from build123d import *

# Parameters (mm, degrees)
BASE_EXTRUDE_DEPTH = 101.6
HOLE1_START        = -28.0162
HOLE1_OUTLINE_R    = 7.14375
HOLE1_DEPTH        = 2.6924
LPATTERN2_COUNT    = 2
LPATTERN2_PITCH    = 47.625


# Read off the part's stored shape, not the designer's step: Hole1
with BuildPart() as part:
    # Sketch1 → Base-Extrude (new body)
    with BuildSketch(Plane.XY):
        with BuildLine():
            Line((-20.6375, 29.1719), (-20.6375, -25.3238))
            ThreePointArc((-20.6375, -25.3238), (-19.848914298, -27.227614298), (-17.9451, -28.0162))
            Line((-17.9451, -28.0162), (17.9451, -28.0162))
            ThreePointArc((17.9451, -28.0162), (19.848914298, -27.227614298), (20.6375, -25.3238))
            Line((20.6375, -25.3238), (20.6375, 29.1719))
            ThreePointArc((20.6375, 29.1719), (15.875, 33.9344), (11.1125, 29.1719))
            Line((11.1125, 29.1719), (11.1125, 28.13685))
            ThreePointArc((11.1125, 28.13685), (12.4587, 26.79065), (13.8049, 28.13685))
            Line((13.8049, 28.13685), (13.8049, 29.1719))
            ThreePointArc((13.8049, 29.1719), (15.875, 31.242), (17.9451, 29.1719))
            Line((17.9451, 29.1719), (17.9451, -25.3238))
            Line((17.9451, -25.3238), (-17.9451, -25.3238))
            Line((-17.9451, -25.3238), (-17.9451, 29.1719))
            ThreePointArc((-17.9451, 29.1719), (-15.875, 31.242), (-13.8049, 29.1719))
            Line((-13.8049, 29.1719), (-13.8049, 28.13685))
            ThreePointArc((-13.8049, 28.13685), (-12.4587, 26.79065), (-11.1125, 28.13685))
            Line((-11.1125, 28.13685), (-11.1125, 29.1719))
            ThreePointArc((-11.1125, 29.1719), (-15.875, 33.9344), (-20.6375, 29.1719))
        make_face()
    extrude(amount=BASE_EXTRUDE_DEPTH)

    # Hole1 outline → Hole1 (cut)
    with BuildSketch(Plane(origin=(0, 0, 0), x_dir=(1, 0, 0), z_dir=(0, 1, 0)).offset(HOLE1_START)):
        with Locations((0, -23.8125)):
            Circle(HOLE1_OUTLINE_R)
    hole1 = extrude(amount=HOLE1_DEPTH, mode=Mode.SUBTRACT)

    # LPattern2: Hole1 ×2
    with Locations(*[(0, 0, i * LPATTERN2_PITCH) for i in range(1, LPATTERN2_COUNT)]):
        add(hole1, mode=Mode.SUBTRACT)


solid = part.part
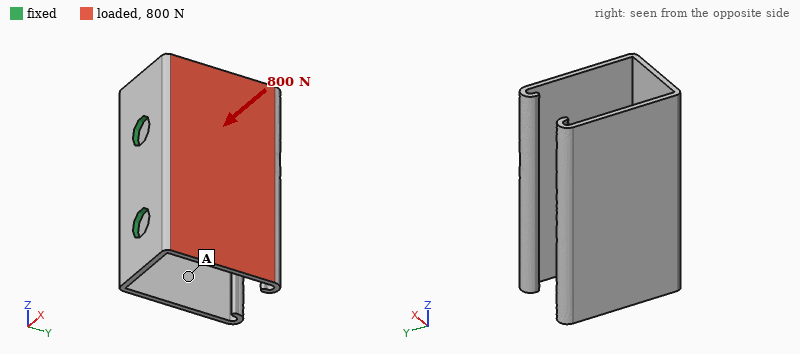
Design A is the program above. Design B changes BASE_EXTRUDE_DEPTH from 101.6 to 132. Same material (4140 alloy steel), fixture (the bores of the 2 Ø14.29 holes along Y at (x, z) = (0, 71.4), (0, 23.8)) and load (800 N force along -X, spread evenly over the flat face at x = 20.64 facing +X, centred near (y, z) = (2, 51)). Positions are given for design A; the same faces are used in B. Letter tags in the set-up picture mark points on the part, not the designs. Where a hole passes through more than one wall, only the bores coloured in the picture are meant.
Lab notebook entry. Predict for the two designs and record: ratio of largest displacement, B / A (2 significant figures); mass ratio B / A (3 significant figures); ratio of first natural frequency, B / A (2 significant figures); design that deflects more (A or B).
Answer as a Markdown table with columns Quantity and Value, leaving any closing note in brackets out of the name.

| Quantity | Value |
|---|---|
| ratio of largest displacement, B / A | 0.85 |
| mass ratio B / A | 1.30 |
| ratio of first natural frequency, B / A | 0.95 |
| design that deflects more | A |
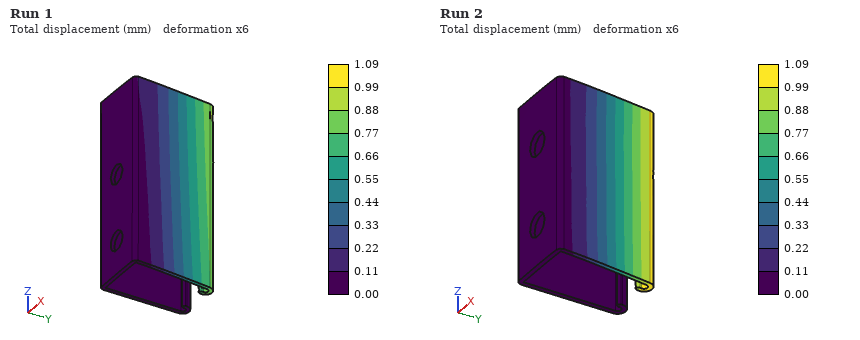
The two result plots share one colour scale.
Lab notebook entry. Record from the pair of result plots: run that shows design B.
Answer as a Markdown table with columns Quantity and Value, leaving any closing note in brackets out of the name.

| Quantity | Value |
|---|---|
| run that shows design B | Run 1 |
